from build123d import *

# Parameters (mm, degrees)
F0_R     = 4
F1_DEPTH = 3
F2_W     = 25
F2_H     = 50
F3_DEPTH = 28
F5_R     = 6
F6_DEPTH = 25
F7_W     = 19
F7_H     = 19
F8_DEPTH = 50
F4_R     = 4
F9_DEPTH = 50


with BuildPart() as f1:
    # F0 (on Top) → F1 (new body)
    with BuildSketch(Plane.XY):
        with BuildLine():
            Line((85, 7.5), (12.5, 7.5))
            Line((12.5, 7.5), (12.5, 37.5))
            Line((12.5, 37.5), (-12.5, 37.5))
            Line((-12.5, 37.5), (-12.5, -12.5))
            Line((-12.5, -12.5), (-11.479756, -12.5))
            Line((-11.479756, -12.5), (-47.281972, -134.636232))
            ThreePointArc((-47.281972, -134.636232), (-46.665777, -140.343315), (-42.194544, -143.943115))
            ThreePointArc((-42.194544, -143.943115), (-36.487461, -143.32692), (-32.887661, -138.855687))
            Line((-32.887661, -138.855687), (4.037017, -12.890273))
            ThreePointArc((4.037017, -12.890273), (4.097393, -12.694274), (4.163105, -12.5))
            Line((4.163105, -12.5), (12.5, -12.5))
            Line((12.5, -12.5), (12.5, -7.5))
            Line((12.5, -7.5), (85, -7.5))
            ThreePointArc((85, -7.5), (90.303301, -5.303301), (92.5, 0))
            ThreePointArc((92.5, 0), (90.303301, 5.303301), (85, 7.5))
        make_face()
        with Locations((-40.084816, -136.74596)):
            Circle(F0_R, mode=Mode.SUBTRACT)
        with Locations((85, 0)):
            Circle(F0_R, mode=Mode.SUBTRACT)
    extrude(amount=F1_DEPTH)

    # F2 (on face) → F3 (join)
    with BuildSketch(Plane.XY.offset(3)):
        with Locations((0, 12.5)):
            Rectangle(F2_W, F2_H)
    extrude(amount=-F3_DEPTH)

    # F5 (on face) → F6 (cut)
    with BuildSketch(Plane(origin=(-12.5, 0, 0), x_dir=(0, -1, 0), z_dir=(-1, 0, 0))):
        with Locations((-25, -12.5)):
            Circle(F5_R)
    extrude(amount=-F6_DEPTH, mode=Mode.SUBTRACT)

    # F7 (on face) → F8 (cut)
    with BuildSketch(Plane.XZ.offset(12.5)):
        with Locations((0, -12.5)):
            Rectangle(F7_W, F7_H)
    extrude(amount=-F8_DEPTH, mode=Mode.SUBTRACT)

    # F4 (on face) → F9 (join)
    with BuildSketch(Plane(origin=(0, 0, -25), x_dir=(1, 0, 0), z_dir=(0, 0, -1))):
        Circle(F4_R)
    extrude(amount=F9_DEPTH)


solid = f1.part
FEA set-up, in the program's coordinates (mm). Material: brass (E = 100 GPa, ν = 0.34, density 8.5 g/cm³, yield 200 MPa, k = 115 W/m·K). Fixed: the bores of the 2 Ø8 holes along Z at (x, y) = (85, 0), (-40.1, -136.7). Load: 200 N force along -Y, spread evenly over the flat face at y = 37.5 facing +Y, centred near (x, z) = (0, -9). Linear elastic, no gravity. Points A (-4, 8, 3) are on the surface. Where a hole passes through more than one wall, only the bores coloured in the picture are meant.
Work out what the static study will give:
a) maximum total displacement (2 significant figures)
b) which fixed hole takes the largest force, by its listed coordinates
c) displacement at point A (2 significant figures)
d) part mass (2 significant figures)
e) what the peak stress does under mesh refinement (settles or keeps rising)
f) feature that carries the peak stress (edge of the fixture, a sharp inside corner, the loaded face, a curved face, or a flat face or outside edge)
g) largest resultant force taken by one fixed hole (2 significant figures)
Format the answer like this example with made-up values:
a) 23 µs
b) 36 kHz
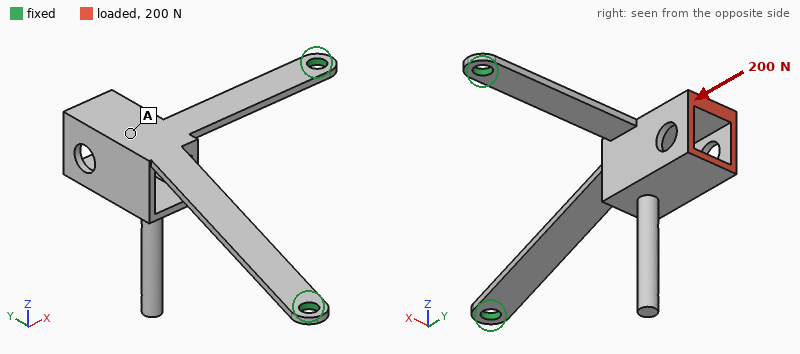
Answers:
a) 1.4 mm
b) (-40.1, -136.7)
c) 0.60 mm
d) 240 g
e) keeps rising
f) edge of the fixture
g) 200 N
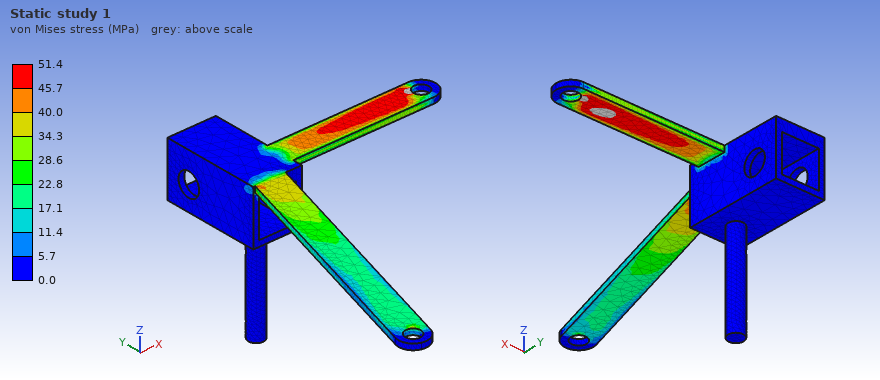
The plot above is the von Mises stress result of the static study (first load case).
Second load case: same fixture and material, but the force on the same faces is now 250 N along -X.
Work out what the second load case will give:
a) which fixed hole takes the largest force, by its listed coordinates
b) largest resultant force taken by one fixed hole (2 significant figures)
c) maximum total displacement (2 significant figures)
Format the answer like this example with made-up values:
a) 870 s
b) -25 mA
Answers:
a) (85, 0)
b) 280 N
c) 2.1 mm
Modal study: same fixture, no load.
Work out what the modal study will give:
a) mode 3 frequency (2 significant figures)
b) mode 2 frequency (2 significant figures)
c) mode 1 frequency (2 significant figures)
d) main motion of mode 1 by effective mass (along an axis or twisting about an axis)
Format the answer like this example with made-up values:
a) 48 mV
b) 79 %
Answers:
a) 300 Hz
b) 200 Hz
c) 68 Hz
d) along Z
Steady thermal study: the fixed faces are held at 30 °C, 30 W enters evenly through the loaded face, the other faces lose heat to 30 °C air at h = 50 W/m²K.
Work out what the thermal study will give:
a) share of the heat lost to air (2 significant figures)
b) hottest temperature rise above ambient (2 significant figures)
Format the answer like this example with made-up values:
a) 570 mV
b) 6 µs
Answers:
a) 91 %
b) 63 K
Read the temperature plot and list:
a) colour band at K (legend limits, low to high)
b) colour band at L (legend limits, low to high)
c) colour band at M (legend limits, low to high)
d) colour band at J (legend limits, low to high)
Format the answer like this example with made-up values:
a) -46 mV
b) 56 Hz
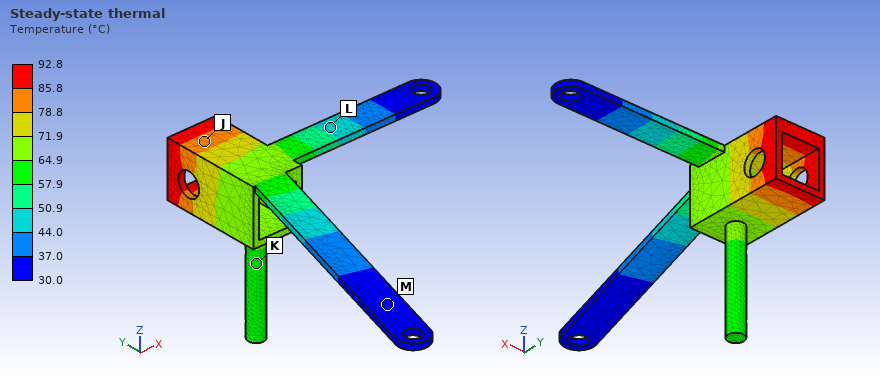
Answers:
a) 57.9 to 64.9 °C
b) 44.0 to 50.9 °C
c) 30.0 to 37.0 °C
d) 78.8 to 85.8 °C
